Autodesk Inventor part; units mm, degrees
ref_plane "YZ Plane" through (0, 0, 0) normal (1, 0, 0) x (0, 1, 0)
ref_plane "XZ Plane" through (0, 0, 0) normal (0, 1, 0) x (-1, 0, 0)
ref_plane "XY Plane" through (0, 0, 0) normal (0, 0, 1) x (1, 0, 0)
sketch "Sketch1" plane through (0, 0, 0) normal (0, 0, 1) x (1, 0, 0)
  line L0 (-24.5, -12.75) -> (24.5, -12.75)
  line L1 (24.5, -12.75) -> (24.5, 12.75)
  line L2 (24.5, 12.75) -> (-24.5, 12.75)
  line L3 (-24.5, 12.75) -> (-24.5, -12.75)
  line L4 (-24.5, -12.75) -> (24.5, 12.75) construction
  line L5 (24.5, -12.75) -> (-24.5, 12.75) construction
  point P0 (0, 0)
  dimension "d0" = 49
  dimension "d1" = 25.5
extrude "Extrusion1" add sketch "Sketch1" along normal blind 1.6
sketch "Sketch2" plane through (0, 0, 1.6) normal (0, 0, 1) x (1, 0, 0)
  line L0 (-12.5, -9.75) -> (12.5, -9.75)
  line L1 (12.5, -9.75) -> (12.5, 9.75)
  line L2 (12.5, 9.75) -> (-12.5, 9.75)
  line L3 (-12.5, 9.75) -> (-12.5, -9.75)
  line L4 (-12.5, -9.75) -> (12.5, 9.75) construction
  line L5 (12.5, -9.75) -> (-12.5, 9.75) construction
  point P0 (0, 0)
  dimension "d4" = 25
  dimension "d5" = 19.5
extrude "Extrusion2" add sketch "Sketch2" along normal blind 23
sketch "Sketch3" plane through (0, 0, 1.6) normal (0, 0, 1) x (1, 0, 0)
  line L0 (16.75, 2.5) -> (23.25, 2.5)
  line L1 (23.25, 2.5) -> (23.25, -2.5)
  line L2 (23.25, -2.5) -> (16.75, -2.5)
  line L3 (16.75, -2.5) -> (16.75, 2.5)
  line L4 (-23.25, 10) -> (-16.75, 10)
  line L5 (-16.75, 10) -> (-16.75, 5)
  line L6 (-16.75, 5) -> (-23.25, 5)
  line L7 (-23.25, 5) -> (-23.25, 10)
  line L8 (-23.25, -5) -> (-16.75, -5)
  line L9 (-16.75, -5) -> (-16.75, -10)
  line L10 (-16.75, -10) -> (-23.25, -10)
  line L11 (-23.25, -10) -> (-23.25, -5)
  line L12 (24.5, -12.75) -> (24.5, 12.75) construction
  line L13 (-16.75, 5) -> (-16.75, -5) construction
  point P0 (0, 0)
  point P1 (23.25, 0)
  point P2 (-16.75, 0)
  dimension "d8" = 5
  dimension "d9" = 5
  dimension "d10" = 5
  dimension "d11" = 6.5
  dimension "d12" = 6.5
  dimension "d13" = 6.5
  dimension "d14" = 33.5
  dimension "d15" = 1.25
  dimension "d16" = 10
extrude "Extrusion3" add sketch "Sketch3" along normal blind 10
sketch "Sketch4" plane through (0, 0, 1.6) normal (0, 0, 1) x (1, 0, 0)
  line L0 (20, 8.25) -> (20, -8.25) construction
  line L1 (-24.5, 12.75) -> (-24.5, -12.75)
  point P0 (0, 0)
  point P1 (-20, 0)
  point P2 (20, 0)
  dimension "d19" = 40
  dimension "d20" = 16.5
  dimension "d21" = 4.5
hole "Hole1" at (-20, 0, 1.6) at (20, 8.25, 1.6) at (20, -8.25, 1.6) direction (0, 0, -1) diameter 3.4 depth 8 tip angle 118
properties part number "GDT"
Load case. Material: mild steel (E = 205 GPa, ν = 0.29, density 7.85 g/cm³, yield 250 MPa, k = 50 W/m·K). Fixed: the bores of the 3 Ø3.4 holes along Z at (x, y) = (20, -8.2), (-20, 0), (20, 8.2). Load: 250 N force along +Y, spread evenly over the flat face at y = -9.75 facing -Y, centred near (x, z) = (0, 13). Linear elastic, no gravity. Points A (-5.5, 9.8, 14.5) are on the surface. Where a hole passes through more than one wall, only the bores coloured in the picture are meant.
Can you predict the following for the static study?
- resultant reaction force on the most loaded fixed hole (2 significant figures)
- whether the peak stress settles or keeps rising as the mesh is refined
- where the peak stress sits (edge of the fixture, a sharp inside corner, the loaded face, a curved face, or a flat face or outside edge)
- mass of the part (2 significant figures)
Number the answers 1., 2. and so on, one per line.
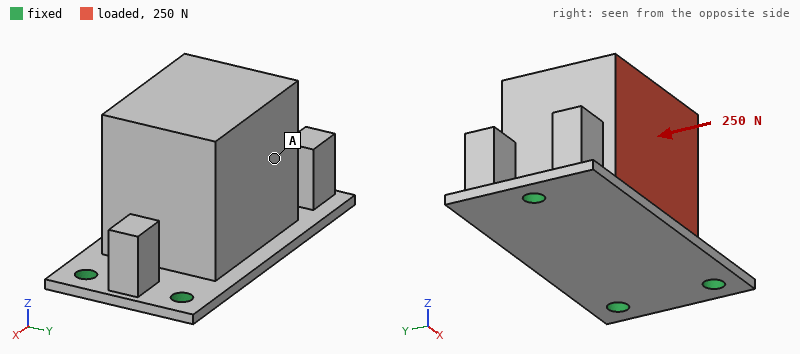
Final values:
1. 210 N
2. keeps rising
3. edge of the fixture
4. 110 g
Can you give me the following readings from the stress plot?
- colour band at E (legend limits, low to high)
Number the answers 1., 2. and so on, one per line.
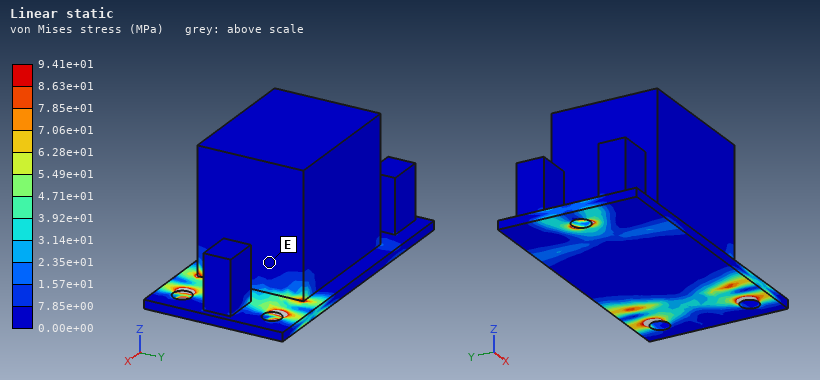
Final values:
1. 0.00e+00 to 7.85e+00 MPa
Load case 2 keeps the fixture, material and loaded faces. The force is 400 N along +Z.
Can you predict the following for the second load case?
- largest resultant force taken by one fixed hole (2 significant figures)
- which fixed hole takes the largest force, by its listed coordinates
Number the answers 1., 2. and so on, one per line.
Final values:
1. 320 N
2. (20, -8.2)
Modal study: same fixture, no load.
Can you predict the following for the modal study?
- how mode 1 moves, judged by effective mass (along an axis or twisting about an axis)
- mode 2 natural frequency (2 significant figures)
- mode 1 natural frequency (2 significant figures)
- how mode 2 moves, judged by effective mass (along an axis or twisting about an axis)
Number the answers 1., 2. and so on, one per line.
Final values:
1. along Y
2. 3500 Hz
3. 1900 Hz
4. along Z
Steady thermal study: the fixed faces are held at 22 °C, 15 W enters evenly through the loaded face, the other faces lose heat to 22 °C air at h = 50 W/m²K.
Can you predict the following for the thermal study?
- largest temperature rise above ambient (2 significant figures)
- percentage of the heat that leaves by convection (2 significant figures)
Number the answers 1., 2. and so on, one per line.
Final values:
1. 37 K
2. 35 %
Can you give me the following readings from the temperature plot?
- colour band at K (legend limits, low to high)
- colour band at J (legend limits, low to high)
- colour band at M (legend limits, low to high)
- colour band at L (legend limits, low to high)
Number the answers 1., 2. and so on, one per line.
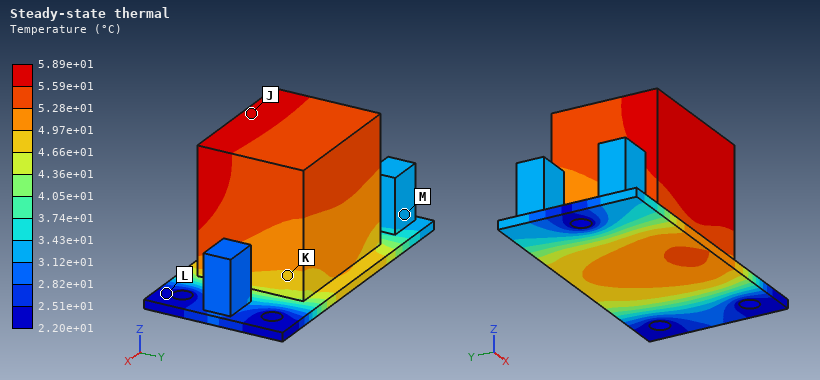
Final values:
1. 4.66e+01 to 4.97e+01 °C
2. 5.59e+01 to 5.89e+01 °C
3. 3.12e+01 to 3.43e+01 °C
4. 2.20e+01 to 2.51e+01 °C
